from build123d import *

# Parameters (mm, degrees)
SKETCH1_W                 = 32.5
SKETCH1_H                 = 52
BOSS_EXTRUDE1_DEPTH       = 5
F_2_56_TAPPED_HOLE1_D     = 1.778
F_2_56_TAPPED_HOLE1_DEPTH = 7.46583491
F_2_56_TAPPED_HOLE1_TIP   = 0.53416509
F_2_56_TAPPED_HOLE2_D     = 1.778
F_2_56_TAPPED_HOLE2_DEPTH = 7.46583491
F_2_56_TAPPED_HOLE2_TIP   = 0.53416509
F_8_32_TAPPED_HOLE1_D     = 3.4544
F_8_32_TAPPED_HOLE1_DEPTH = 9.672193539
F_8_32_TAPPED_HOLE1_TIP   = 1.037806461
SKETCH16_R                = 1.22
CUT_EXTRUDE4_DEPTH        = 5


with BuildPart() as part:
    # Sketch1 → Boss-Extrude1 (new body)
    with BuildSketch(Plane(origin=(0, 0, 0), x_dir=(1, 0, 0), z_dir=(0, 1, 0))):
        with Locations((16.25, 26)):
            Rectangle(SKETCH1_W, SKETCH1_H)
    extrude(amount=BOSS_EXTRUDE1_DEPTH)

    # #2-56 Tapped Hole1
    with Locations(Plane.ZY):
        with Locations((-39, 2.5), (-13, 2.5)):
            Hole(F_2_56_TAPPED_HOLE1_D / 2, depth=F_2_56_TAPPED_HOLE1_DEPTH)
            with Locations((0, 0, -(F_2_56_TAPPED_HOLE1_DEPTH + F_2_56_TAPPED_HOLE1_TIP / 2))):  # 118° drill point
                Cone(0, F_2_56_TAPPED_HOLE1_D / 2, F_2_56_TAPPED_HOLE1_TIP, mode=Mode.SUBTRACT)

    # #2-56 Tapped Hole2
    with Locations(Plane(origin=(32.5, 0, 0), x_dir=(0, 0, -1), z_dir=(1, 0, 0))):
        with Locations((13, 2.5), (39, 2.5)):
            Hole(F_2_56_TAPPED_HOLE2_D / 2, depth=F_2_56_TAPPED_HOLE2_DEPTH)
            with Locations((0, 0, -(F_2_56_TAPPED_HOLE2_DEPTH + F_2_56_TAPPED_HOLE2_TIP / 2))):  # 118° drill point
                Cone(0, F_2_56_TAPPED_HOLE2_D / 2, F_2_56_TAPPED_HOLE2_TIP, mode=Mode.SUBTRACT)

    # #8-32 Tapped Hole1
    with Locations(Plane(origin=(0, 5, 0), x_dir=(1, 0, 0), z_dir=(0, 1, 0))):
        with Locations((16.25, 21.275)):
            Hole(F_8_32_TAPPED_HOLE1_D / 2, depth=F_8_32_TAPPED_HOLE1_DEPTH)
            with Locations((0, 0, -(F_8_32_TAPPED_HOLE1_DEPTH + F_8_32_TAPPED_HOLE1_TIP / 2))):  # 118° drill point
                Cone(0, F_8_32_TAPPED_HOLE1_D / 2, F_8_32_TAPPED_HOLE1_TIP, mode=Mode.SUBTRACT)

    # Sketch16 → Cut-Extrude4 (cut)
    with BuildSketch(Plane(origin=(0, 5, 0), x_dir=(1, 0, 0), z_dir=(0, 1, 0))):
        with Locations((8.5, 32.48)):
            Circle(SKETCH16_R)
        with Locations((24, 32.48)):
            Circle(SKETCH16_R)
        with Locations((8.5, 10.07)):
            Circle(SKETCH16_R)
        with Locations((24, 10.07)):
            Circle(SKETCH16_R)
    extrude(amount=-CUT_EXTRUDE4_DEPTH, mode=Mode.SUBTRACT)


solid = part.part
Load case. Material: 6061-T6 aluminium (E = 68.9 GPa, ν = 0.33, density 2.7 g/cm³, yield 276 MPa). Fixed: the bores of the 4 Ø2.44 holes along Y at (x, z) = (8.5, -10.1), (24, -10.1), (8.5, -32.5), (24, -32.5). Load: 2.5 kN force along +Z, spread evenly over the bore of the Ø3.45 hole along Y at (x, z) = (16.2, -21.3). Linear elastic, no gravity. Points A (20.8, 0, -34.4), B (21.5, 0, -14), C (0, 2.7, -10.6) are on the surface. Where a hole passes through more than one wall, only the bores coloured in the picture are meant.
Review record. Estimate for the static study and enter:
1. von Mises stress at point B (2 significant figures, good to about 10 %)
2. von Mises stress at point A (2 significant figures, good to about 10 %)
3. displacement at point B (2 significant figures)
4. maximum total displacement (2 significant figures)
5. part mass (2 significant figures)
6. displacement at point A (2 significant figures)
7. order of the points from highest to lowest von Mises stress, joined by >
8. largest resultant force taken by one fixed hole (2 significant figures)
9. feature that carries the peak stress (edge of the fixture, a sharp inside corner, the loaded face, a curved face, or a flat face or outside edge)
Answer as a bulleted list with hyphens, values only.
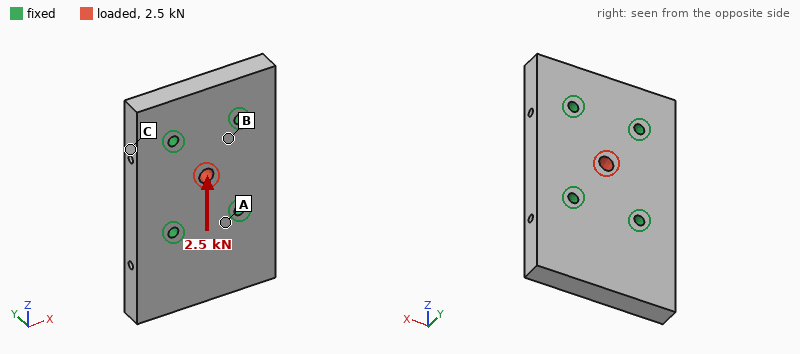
- 19 MPa
- 8.8 MPa
- 1.2 µm
- 4.5 µm
- 22 g
- 0.75 µm
- B > A > C
- 660 N
- the loaded face
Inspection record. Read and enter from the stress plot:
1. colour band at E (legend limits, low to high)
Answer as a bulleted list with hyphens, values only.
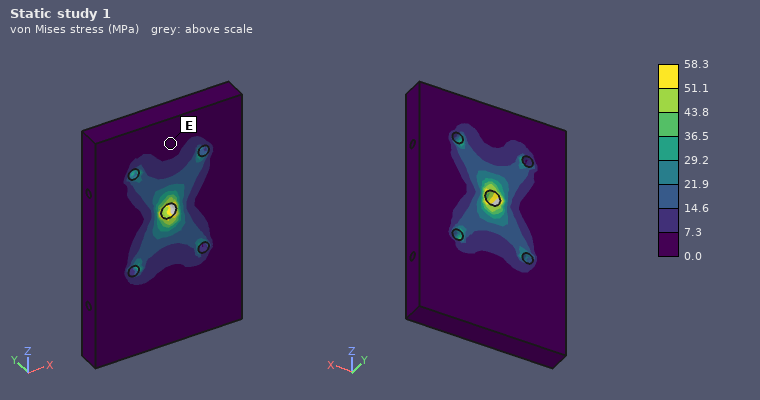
- 0.0 to 7.3 MPa
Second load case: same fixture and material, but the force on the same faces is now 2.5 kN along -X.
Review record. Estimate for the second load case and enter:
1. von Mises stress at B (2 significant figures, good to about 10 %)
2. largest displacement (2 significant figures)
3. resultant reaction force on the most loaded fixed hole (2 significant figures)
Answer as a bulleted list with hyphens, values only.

- 21 MPa
- 5.8 µm
- 680 N
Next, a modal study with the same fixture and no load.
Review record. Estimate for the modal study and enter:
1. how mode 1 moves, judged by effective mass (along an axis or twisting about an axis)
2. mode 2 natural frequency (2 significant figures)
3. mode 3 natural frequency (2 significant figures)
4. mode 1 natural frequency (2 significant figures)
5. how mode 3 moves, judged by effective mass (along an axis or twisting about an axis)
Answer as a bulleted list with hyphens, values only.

- along Y
- 15 kHz
- 26 kHz
- 9400 Hz
- along X
